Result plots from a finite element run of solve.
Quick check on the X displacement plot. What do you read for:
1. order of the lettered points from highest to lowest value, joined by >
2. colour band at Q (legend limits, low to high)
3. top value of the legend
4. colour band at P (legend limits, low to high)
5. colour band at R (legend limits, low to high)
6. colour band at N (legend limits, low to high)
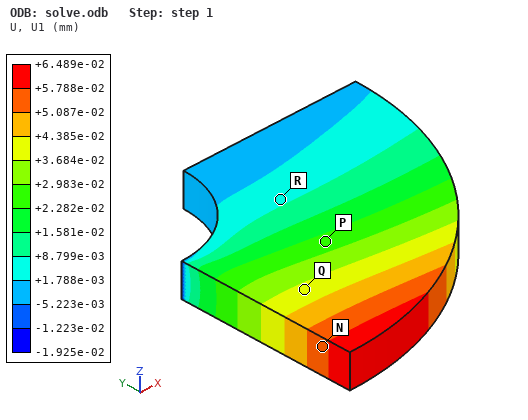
N > Q > P > R
+3.684e-02 to +4.385e-02 mm
+6.489e-02 mm
+2.282e-02 to +2.983e-02 mm
+1.788e-03 to +8.799e-03 mm
+5.087e-02 to +5.788e-02 mm
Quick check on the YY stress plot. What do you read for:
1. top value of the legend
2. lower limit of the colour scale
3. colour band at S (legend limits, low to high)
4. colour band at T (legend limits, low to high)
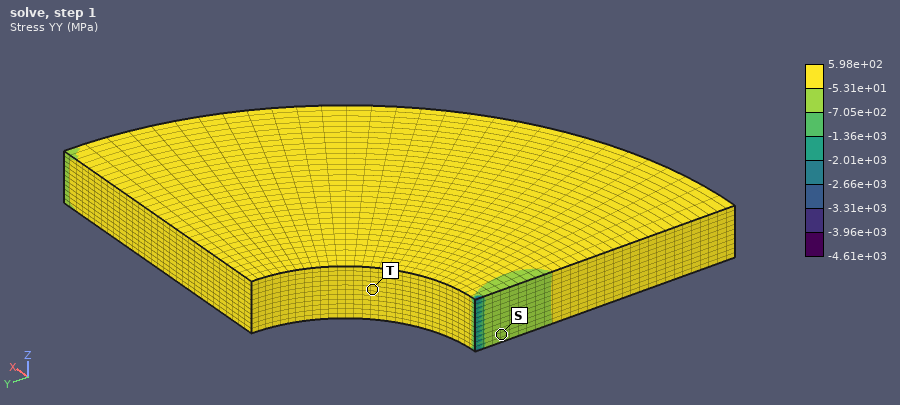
5.98e+02 MPa
-4.61e+03 MPa
-7.05e+02 to -5.31e+01 MPa
-5.31e+01 to 5.98e+02 MPa
